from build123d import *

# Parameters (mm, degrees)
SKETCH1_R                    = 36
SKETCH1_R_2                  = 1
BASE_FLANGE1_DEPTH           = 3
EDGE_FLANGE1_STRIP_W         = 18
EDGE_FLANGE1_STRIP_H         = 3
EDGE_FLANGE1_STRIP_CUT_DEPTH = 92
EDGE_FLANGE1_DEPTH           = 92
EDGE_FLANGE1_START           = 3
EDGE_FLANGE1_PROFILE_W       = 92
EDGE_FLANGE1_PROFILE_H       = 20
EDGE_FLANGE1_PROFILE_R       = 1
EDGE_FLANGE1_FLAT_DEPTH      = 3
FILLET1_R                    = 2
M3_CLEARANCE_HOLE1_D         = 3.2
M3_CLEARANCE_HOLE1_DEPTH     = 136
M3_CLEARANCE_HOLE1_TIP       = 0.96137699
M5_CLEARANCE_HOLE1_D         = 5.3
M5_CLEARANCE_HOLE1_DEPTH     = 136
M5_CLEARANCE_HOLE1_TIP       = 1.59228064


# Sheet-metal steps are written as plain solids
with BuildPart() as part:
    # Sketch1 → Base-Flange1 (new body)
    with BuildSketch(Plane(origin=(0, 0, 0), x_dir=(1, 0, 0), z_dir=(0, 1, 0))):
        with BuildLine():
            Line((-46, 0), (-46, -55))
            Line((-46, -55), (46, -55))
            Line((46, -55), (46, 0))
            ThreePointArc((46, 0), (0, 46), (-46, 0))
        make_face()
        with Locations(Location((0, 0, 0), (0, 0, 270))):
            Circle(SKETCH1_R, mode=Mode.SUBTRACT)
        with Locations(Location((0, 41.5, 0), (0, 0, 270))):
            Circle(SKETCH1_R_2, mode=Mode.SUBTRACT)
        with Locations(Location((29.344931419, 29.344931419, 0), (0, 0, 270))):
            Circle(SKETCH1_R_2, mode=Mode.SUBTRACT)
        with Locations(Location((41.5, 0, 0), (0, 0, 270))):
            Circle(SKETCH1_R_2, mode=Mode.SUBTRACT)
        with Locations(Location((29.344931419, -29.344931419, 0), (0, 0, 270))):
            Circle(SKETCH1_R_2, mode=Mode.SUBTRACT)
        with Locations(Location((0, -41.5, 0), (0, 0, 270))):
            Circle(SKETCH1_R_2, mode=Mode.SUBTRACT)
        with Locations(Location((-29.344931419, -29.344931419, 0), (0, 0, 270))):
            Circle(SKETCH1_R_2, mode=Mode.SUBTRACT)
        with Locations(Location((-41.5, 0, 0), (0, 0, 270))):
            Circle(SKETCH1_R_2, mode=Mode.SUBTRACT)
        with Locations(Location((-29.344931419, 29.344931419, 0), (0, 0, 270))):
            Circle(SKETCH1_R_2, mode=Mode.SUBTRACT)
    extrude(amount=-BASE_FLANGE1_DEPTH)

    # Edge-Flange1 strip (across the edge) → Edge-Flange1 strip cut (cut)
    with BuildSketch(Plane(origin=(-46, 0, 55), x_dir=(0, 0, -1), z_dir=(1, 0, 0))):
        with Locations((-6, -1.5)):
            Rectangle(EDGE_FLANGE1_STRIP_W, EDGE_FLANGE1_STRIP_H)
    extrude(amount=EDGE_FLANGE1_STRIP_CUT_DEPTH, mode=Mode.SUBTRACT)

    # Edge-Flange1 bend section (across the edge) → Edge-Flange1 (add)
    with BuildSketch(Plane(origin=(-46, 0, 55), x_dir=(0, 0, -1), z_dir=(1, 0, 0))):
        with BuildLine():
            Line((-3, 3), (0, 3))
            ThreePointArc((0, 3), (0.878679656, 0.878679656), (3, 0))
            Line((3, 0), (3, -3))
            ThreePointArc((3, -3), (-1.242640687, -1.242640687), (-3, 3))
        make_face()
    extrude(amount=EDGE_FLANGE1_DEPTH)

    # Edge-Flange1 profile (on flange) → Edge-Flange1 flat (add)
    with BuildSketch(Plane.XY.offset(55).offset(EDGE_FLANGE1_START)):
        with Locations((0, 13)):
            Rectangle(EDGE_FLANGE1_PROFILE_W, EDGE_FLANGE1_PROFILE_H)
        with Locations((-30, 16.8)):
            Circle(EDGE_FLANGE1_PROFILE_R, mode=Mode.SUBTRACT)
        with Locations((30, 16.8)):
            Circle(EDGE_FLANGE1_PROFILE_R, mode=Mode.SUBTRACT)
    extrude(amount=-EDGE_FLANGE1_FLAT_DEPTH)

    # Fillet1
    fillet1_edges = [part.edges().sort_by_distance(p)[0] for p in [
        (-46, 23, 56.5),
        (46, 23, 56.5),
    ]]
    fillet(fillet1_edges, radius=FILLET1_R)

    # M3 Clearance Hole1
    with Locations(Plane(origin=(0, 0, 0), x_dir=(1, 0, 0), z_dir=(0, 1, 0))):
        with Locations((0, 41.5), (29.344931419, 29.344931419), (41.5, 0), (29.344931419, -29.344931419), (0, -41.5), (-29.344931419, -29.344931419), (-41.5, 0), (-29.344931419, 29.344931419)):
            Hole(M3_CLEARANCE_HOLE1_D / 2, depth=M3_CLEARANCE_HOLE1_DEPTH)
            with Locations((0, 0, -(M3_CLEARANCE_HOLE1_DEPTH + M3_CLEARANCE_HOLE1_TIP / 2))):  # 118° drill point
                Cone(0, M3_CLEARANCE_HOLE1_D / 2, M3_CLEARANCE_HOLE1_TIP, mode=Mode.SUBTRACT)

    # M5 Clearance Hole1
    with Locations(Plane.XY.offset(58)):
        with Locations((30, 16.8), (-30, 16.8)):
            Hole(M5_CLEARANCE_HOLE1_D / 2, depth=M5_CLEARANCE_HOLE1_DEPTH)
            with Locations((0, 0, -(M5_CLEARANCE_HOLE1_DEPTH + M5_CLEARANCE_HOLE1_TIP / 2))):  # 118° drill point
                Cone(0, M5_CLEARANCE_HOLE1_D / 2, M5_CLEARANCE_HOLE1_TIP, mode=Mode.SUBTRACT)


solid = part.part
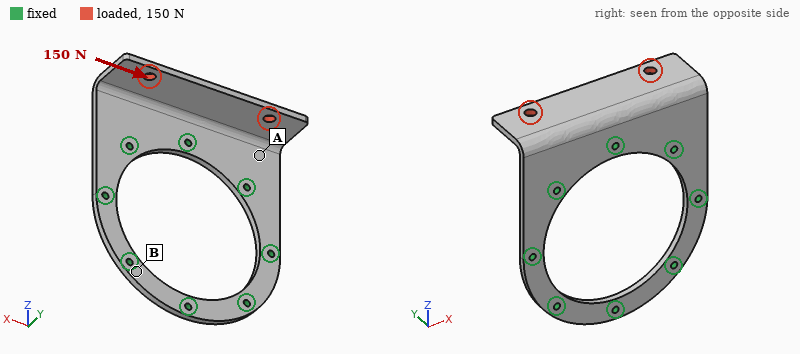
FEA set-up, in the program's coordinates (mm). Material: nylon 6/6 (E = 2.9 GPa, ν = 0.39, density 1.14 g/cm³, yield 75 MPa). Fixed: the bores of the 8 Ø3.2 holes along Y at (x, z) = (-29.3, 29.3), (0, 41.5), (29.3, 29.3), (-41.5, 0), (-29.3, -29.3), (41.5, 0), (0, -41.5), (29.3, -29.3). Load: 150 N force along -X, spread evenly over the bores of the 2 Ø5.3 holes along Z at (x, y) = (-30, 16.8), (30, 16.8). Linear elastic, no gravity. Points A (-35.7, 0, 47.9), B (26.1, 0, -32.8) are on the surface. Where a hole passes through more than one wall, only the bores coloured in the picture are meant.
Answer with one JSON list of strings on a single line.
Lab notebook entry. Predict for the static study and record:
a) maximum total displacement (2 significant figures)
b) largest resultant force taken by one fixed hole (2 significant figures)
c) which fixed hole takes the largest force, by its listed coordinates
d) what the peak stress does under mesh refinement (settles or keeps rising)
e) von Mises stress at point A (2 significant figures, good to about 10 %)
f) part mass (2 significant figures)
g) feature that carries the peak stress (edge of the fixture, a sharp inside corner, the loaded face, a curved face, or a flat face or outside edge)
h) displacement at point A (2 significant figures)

["1.5 mm", "95 N", "(0, 41.5)", "keeps rising", "4.5 MPa", "22 g", "edge of the fixture", "0.54 mm"]
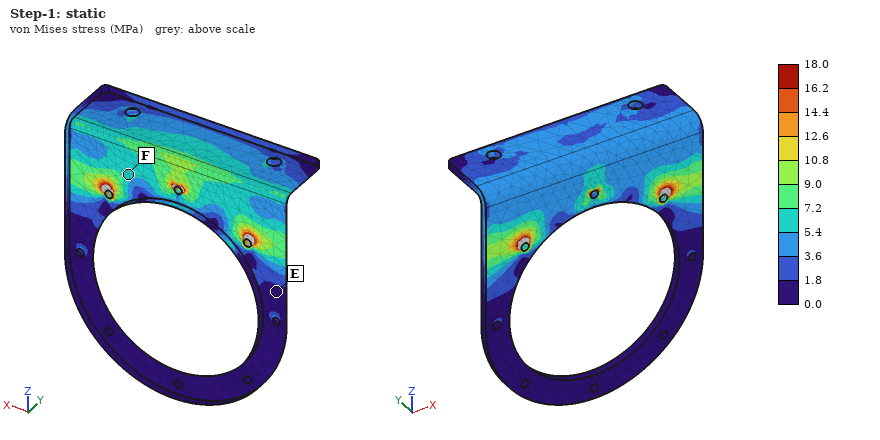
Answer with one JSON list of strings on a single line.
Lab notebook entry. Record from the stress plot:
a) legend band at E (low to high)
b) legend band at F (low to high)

["0.0 to 1.8 MPa", "5.4 to 7.2 MPa"]
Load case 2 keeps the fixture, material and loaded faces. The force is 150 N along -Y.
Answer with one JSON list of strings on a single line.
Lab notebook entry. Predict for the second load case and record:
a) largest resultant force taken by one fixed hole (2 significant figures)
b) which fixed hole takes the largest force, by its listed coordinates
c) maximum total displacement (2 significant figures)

["150 N", "(0, 41.5)", "1.5 mm"]
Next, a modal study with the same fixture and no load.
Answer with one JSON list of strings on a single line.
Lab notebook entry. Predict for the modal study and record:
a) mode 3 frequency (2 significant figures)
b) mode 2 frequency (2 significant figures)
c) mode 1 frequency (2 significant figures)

["1300 Hz", "550 Hz", "550 Hz"]
